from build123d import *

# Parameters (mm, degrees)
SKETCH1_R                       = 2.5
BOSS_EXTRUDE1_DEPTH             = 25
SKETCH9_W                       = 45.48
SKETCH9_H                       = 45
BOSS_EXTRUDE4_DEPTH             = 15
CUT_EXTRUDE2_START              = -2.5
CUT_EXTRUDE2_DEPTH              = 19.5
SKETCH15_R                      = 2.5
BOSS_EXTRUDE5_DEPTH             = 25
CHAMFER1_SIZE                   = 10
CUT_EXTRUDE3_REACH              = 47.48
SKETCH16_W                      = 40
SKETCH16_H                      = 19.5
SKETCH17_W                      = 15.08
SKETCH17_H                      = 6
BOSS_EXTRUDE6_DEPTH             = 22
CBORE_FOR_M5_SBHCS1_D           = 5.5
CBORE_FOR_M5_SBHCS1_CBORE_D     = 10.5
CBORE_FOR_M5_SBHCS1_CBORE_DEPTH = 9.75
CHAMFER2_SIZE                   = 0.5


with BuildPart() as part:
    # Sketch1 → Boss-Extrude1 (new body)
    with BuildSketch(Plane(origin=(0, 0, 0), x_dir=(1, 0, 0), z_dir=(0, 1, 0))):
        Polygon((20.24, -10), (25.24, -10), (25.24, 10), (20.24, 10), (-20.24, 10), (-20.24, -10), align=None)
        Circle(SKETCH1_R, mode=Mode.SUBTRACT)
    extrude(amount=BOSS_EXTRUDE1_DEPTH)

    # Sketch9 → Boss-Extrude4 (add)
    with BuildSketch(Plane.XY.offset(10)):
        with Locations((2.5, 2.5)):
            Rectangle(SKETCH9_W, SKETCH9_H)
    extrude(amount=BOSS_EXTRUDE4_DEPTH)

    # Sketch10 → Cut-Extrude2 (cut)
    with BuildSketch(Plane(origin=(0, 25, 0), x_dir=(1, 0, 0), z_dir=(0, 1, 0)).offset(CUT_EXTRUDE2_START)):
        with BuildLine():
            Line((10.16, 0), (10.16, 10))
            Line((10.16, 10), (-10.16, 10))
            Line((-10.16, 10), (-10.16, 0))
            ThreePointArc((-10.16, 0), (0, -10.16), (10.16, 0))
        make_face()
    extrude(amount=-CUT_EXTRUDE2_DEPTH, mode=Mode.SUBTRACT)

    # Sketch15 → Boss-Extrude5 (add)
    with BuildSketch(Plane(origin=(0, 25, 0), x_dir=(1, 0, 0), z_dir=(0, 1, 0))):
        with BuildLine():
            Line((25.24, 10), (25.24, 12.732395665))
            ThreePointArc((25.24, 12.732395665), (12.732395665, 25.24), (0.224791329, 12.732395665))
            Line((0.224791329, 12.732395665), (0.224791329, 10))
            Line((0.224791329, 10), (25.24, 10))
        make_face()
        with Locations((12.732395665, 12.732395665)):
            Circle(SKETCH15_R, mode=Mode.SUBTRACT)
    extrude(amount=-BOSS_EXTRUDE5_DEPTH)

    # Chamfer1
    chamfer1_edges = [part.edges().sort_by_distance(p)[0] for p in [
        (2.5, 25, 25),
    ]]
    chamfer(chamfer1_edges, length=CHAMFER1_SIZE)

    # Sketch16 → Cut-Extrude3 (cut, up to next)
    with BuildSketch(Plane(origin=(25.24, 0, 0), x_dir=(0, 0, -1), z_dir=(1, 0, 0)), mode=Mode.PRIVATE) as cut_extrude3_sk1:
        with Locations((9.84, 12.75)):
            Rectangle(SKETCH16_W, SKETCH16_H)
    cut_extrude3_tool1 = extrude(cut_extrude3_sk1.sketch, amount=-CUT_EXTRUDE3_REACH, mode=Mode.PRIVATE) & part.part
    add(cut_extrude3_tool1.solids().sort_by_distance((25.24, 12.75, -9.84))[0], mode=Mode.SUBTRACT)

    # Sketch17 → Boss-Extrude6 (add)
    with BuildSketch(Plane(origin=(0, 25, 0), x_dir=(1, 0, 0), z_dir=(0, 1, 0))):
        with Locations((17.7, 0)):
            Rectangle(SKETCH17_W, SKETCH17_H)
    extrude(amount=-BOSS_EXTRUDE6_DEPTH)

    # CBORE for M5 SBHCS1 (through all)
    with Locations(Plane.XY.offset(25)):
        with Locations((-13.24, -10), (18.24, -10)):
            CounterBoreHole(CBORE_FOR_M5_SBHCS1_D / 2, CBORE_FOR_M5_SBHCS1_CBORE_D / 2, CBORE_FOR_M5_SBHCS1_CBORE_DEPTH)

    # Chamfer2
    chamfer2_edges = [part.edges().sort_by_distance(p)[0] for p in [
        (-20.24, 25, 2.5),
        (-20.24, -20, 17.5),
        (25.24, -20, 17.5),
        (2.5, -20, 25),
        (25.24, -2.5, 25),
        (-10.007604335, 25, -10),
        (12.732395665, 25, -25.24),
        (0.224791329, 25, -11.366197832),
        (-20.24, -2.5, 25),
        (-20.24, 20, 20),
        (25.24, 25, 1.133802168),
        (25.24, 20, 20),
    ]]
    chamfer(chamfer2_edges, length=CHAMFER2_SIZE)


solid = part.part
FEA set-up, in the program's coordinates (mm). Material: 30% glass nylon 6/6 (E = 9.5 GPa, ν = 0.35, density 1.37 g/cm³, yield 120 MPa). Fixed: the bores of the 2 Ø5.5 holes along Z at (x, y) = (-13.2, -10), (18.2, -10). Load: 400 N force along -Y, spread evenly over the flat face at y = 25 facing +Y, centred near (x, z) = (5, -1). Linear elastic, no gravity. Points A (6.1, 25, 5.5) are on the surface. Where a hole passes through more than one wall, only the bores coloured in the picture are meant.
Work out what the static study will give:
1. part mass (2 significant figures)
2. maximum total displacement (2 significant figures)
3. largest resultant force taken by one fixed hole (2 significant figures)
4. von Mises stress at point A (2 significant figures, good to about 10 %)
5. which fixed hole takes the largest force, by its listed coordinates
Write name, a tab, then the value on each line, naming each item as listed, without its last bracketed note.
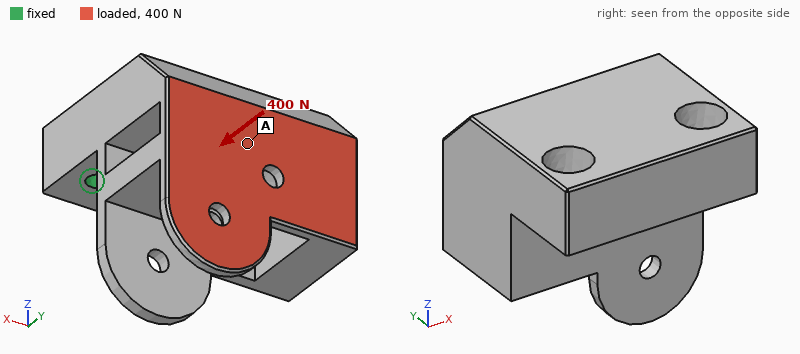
part mass	53 g
maximum total displacement	0.82 mm
largest resultant force taken by one fixed hole	230 N
von Mises stress at point A	4.3 MPa
which fixed hole takes the largest force, by its listed coordinates	(18.2, -10)
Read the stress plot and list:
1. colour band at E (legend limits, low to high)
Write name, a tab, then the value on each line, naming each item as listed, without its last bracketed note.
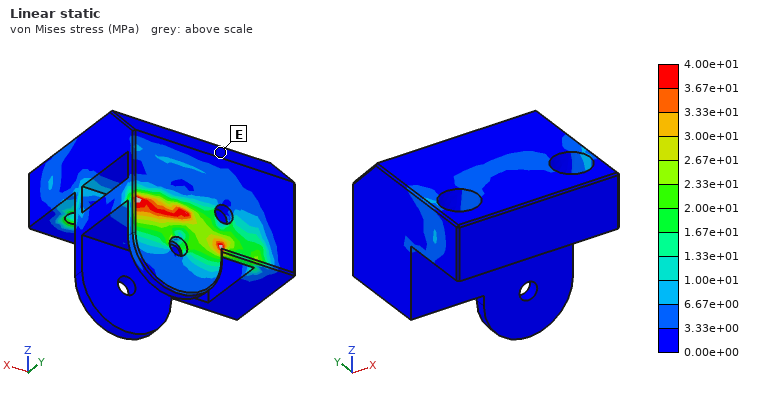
colour band at E	0.00e+00 to 3.33e+00 MPa
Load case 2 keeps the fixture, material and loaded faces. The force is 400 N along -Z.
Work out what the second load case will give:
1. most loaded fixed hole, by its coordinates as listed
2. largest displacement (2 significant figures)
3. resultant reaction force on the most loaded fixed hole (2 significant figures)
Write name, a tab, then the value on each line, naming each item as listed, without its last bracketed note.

most loaded fixed hole, by its coordinates as listed	(18.2, -10)
largest displacement	0.47 mm
resultant reaction force on the most loaded fixed hole	230 N
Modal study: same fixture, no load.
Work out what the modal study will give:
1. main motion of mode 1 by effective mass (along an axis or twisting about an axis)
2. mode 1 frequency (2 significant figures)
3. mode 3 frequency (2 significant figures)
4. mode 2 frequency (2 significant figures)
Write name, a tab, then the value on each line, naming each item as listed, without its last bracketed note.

main motion of mode 1 by effective mass	along Z
mode 1 frequency	1400 Hz
mode 3 frequency	2600 Hz
mode 2 frequency	2300 Hz
